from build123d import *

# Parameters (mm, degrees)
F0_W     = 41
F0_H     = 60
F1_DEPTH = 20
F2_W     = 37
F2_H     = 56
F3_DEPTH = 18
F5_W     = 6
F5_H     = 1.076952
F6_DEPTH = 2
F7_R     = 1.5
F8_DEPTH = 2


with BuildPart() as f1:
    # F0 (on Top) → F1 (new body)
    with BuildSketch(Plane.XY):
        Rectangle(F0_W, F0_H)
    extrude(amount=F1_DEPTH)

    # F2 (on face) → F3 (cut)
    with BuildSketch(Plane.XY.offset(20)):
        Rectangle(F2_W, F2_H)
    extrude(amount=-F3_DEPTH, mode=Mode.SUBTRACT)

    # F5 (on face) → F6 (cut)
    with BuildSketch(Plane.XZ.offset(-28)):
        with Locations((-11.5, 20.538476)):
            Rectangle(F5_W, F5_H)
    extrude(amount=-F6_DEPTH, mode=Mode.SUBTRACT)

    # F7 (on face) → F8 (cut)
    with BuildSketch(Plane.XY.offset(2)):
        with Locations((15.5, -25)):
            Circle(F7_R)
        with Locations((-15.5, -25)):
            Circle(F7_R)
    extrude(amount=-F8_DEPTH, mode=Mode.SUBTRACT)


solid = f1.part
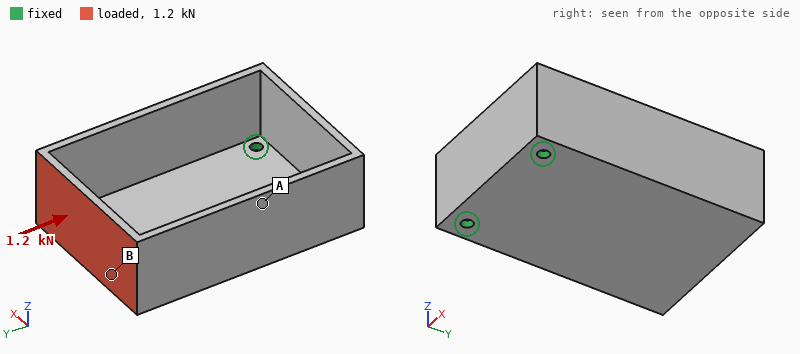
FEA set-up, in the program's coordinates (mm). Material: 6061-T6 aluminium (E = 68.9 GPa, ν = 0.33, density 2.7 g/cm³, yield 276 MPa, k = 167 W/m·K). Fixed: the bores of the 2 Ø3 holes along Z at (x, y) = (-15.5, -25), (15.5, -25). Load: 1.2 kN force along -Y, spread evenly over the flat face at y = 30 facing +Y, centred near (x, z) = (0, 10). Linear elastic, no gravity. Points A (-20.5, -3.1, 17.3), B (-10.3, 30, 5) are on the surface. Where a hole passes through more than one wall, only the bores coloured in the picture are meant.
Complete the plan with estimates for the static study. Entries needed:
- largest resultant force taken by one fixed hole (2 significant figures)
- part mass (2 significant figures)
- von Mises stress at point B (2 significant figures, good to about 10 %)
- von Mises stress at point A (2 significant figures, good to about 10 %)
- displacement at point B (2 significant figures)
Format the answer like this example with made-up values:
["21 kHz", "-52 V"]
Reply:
["600 N", "32 g", "72 MPa", "27 MPa", "0.59 mm"]
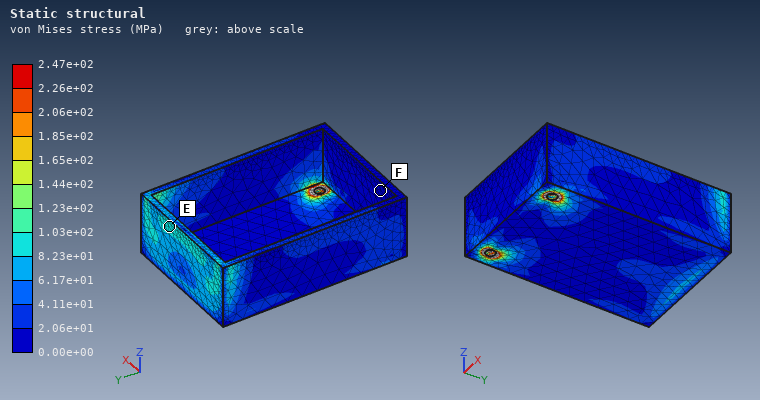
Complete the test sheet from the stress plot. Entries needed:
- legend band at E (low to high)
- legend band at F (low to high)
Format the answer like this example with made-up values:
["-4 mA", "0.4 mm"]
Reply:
["8.23e+01 to 1.03e+02 MPa", "0.00e+00 to 2.06e+01 MPa"]
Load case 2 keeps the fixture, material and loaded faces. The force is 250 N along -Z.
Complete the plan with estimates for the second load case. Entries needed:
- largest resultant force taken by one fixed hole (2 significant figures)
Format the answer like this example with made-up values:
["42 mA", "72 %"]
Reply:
["140 N"]
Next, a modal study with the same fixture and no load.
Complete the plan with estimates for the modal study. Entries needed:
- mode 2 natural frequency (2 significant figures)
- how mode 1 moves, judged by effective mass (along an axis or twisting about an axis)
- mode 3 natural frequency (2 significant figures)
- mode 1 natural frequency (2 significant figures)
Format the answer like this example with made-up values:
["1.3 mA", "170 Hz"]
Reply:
["1400 Hz", "along Z", "4500 Hz", "840 Hz"]
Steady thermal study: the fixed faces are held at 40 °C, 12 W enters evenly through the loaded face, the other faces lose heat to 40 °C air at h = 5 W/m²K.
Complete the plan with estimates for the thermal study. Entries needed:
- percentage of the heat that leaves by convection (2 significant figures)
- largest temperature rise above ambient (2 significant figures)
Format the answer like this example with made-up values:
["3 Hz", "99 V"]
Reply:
["6.8 %", "32 K"]
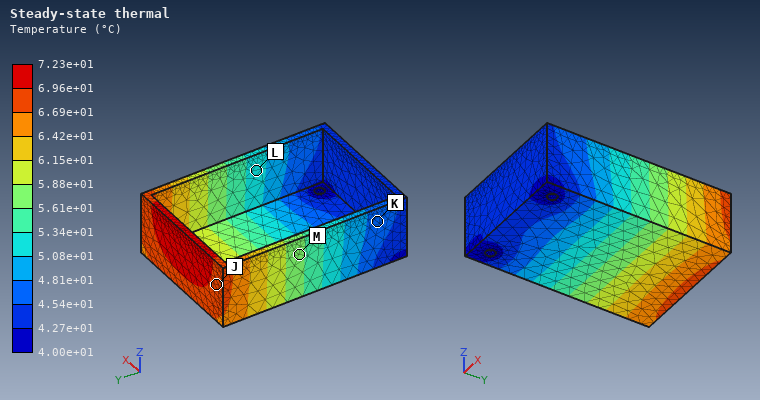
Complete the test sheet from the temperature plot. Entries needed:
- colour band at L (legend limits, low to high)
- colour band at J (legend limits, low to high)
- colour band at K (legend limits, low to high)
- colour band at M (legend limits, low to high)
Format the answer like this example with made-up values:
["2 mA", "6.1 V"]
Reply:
["5.08e+01 to 5.34e+01 °C", "6.69e+01 to 6.96e+01 °C", "4.54e+01 to 4.81e+01 °C", "5.61e+01 to 5.88e+01 °C"]
